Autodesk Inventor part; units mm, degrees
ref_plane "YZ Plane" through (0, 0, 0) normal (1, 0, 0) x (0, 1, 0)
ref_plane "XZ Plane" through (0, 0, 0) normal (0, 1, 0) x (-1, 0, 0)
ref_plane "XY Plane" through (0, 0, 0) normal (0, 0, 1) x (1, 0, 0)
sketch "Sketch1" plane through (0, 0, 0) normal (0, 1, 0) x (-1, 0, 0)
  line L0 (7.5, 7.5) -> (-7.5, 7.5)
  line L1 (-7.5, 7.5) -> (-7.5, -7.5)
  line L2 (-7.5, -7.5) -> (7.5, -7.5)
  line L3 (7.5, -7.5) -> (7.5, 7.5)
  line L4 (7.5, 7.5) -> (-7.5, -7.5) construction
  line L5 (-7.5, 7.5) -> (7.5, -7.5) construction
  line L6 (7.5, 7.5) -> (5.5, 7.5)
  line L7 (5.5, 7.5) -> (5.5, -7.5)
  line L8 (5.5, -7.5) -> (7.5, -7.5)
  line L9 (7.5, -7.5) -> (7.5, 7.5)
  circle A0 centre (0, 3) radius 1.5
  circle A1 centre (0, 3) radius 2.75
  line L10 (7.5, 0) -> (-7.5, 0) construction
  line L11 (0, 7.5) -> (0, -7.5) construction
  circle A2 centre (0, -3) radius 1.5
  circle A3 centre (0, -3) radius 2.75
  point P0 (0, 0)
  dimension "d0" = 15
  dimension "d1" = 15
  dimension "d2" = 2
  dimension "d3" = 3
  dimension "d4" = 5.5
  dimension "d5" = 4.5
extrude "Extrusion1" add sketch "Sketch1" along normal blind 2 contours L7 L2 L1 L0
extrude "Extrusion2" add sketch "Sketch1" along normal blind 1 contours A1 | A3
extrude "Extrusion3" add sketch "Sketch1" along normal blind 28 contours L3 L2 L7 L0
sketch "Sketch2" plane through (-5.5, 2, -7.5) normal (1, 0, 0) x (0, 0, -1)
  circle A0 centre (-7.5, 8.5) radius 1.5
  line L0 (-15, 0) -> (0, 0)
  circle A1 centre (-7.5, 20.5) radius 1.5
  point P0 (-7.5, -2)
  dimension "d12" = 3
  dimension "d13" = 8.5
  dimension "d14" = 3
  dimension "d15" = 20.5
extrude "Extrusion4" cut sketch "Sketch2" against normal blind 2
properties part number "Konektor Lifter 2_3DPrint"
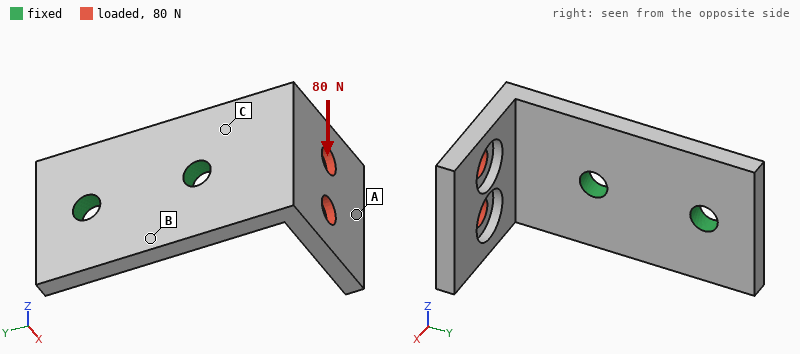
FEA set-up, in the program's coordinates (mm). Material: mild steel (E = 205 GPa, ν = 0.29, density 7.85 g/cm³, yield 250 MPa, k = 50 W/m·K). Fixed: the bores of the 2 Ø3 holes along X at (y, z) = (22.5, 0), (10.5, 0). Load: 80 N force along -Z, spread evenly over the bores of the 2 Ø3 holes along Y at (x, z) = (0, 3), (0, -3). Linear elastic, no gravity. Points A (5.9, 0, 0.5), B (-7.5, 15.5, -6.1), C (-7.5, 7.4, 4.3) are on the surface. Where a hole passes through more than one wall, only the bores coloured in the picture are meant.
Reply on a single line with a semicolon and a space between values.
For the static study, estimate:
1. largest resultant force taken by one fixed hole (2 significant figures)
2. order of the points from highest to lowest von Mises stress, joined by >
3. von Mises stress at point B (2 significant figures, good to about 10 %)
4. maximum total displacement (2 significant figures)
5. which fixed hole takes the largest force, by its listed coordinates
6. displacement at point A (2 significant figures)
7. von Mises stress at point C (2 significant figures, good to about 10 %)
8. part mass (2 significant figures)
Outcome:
120 N; C > B > A; 15 MPa; 21 µm; (10.5, 0); 17 µm; 24 MPa; 8.9 g
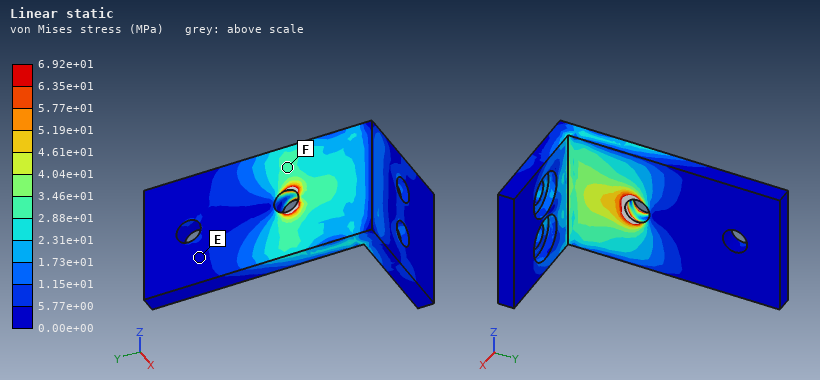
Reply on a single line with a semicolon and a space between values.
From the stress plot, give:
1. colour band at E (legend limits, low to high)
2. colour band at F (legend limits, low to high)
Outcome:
0.00e+00 to 5.77e+00 MPa; 2.88e+01 to 3.46e+01 MPa
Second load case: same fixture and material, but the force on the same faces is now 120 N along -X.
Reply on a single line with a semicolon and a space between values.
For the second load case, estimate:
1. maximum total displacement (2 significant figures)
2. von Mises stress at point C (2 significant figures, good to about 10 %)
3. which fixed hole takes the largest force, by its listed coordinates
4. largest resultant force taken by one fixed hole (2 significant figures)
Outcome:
44 µm; 66 MPa; (10.5, 0); 140 N
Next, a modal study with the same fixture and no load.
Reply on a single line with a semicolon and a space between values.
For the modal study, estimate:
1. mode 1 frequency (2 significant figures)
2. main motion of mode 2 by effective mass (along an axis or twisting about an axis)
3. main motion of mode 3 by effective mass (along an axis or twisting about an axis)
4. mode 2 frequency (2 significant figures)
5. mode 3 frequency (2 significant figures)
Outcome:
4100 Hz; along Z; along X; 6000 Hz; 11 kHz
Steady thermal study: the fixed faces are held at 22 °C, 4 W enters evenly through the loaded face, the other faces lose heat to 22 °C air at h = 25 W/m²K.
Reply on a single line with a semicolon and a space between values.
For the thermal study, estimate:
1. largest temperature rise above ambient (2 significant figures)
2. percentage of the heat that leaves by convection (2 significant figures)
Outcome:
47 K; 15 %
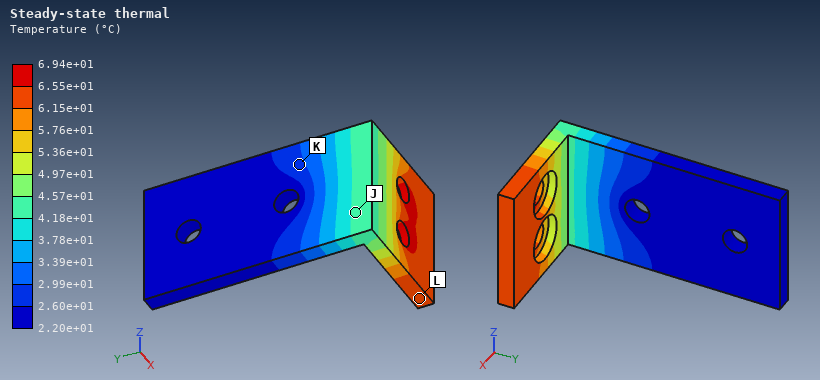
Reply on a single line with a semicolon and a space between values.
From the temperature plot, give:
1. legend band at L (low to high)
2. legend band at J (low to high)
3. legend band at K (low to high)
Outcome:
6.15e+01 to 6.55e+01 °C; 4.18e+01 to 4.57e+01 °C; 2.60e+01 to 2.99e+01 °C
